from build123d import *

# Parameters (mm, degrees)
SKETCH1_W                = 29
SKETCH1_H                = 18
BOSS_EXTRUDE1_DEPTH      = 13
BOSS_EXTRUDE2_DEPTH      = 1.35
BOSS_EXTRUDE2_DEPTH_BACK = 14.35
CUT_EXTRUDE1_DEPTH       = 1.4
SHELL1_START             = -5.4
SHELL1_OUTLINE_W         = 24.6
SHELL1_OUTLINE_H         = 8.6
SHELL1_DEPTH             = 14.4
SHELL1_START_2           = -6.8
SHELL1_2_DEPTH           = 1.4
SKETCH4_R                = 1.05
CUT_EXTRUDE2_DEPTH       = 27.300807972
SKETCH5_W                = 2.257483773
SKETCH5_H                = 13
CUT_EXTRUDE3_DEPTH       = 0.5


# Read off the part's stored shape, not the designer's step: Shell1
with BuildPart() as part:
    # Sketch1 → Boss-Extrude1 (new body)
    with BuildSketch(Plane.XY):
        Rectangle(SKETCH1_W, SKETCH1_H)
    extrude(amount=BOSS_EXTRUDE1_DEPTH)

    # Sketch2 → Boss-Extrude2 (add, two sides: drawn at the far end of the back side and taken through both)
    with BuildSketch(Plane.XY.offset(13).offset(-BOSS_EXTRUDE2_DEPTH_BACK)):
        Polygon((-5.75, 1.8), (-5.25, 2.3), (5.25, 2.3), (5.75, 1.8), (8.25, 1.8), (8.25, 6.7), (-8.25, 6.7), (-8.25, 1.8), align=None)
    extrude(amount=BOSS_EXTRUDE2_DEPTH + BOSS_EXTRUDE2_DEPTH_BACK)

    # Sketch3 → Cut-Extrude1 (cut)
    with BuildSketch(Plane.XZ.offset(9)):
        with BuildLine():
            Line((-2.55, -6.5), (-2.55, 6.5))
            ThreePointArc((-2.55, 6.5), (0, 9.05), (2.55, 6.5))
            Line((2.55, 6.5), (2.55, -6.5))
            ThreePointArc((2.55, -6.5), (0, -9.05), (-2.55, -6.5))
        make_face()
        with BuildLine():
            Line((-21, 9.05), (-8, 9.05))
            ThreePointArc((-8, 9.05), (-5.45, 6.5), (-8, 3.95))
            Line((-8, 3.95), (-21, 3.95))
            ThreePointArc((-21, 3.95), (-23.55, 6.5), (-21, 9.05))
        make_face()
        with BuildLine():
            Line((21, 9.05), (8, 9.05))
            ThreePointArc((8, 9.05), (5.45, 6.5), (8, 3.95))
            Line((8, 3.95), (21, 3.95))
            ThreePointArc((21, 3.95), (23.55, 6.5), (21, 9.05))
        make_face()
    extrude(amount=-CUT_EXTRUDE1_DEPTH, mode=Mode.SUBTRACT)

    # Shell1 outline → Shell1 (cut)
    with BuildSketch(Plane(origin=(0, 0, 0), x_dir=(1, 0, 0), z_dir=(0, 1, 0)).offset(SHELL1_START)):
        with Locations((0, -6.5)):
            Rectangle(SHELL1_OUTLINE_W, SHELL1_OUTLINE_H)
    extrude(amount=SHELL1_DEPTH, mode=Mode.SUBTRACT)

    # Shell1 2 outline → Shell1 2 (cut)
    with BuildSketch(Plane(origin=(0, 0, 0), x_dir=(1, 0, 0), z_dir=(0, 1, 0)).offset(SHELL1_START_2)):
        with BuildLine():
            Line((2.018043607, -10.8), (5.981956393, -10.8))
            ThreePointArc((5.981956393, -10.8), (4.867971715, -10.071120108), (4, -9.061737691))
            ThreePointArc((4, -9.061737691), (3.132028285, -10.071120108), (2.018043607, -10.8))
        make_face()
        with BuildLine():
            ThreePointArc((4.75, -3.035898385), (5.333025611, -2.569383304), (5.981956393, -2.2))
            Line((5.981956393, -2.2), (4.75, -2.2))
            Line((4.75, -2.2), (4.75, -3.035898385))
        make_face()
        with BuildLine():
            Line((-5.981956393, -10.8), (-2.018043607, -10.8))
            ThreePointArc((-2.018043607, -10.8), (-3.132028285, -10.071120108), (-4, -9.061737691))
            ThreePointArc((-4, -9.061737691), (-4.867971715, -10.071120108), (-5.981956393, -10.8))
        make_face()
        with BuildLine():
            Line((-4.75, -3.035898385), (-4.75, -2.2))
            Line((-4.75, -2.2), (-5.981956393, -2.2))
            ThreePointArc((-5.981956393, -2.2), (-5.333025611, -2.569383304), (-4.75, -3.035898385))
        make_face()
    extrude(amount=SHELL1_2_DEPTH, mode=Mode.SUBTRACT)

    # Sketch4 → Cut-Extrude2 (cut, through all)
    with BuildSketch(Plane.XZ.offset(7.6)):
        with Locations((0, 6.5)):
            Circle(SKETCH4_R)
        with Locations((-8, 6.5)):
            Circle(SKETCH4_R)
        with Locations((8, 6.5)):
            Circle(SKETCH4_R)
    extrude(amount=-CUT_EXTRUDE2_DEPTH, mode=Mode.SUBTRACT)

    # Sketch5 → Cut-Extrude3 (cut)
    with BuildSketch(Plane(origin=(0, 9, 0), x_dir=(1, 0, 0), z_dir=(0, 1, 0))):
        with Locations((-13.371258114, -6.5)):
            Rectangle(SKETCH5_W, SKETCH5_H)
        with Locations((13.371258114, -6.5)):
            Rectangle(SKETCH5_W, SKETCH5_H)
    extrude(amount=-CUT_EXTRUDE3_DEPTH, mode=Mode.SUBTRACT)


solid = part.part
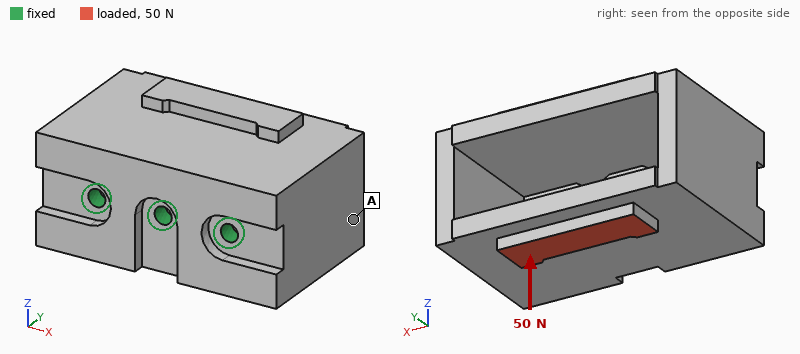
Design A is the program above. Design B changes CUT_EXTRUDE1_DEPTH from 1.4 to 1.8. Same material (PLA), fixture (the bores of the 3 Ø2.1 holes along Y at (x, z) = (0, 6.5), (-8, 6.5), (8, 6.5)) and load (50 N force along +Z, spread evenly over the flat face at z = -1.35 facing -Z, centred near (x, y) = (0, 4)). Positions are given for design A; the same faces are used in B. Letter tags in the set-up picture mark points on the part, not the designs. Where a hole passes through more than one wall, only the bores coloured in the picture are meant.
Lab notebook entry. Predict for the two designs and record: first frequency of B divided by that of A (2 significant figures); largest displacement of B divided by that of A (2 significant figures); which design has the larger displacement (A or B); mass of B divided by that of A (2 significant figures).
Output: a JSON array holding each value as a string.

["0.86", "1.2", "B", "0.99"]
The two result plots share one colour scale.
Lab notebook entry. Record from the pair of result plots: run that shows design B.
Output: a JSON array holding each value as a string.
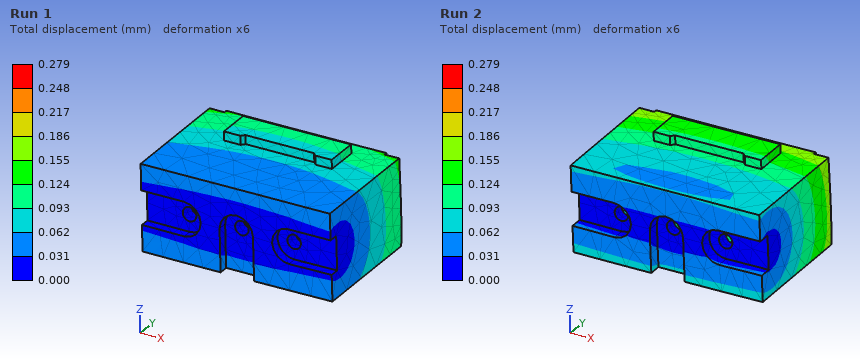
["Run 2"]
